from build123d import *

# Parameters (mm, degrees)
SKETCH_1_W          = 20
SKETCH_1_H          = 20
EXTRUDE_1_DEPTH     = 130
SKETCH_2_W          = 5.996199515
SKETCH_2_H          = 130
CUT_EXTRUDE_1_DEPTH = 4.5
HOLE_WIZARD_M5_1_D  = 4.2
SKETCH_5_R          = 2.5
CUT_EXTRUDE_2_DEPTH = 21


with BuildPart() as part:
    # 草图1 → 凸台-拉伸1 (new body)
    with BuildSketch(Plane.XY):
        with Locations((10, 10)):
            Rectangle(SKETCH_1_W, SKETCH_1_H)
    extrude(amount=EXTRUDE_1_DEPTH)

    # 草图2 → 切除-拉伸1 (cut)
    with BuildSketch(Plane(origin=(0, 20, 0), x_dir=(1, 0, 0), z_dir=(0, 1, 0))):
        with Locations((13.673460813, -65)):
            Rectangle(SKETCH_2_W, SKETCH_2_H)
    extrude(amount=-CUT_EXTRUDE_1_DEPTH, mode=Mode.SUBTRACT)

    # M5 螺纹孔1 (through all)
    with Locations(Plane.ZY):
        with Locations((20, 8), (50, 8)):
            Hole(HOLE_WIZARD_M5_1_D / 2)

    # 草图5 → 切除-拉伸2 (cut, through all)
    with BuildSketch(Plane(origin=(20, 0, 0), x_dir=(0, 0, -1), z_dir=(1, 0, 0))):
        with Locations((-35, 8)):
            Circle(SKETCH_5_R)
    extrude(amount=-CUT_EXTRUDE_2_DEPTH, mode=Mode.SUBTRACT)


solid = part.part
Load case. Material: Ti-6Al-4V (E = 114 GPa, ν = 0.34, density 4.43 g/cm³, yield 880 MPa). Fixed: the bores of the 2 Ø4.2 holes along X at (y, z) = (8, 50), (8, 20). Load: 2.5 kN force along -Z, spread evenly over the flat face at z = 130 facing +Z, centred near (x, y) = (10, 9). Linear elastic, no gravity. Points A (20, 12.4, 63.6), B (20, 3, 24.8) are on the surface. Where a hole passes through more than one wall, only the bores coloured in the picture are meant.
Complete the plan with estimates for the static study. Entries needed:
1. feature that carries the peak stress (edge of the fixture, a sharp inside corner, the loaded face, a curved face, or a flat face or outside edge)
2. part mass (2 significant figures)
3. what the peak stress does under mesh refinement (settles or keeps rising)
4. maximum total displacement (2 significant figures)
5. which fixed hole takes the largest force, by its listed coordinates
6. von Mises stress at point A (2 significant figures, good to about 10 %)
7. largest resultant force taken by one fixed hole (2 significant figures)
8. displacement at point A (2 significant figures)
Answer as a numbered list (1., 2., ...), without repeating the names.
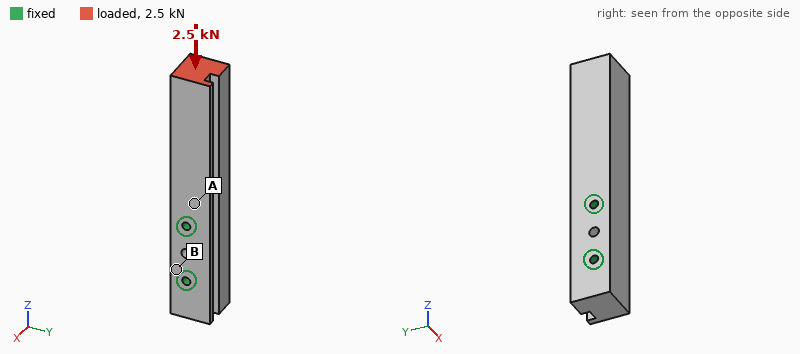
1. edge of the fixture
2. 210 g
3. keeps rising
4. 5.8 µm
5. (8, 50)
6. 6.9 MPa
7. 2.2 kN
8. 1.1 µm
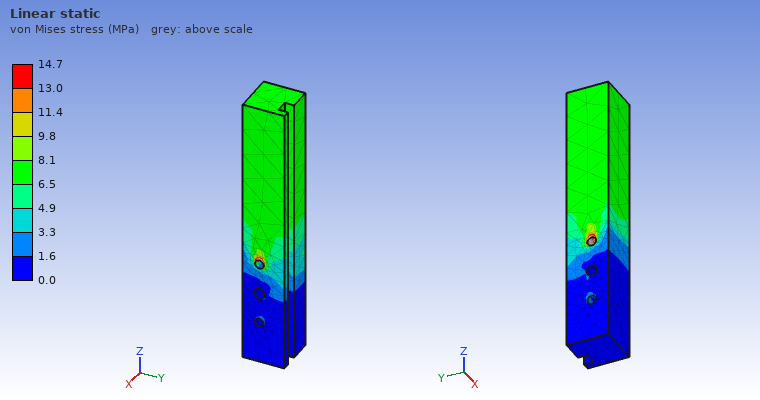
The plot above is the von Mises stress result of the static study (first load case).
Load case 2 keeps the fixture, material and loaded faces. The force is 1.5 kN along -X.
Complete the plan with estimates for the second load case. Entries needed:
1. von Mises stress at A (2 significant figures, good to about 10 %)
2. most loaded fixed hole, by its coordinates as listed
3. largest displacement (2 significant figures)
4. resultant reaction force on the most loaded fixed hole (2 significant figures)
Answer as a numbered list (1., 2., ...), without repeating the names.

1. 82 MPa
2. (8, 50)
3. 0.21 mm
4. 2.3 kN
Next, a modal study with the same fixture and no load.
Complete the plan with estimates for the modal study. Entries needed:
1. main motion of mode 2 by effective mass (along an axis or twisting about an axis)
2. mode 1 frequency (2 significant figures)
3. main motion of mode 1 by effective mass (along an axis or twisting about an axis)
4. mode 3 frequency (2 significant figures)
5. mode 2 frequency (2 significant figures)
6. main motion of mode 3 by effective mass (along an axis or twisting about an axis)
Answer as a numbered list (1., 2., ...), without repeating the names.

1. along X
2. 2000 Hz
3. along Y
4. 8000 Hz
5. 2400 Hz
6. twisting about Z
